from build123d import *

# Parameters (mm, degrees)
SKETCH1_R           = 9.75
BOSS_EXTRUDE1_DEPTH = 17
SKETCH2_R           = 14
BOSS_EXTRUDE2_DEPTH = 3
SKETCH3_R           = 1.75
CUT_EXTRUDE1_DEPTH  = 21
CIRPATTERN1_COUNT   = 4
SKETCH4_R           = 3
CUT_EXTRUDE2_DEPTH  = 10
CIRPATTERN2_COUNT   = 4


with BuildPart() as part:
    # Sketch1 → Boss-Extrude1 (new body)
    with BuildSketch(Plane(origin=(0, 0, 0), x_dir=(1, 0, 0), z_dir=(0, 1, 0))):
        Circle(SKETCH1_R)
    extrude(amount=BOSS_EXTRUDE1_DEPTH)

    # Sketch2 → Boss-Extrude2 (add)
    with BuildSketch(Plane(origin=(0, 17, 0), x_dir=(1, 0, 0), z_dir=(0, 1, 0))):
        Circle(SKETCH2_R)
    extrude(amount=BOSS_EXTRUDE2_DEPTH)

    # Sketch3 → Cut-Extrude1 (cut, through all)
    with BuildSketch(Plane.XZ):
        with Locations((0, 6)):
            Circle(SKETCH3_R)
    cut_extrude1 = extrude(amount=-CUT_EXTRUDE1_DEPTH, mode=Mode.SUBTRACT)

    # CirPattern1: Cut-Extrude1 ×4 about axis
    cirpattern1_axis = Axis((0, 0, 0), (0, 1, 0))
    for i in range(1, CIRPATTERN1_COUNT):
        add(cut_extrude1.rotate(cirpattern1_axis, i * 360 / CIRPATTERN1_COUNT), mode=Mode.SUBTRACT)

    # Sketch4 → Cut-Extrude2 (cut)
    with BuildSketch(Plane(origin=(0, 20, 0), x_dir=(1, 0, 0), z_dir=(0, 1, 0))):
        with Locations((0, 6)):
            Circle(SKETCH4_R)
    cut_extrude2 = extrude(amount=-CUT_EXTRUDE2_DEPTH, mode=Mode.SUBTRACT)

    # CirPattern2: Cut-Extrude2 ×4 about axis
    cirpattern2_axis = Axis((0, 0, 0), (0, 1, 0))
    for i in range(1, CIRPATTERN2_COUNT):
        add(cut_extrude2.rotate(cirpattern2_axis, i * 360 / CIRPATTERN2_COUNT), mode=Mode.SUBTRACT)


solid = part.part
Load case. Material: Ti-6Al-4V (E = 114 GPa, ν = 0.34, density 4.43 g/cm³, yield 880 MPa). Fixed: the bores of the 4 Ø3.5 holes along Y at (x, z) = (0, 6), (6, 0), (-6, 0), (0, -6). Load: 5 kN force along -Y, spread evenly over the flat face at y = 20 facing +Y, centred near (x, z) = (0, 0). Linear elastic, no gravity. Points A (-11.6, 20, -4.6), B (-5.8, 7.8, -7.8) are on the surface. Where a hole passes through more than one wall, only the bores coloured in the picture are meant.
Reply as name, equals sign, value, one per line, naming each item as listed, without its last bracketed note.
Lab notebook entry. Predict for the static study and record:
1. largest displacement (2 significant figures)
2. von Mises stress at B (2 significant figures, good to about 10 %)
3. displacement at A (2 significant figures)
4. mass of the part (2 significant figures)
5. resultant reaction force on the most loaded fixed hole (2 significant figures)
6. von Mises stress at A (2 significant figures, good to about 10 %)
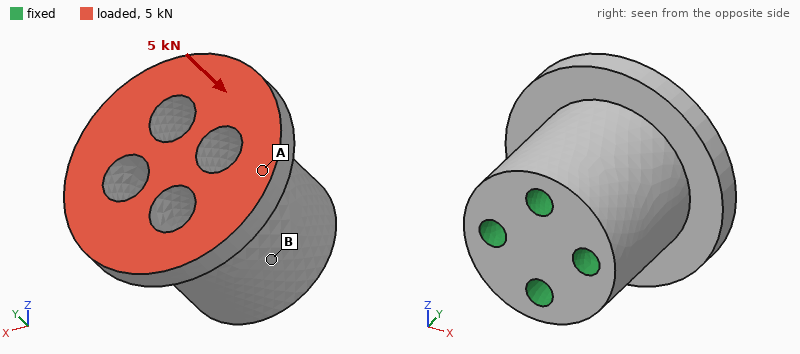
largest displacement = 14 µm
von Mises stress at B = 16 MPa
displacement at A = 11 µm
mass of the part = 24 g
resultant reaction force on the most loaded fixed hole = 1.3 kN
von Mises stress at A = 40 MPa
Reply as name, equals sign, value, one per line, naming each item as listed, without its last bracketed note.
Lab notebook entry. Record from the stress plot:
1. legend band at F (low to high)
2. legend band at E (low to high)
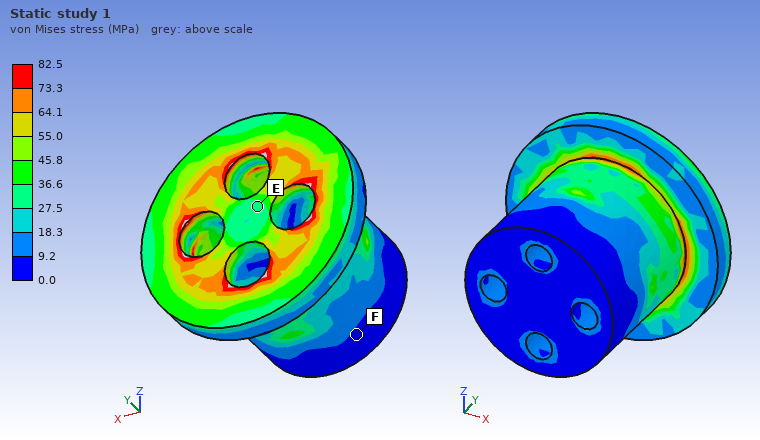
legend band at F = 0.0 to 9.2 MPa
legend band at E = 27.5 to 36.6 MPa
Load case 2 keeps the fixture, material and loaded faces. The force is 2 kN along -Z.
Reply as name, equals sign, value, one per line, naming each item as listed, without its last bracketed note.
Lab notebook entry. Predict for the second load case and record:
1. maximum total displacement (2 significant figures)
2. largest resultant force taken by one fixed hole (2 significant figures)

maximum total displacement = 14 µm
largest resultant force taken by one fixed hole = 1.4 kN
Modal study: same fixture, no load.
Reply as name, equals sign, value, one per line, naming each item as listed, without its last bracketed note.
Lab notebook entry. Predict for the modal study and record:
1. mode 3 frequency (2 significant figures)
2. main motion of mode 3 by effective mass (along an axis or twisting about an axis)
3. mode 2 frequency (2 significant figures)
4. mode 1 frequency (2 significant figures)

mode 3 frequency = 31 kHz
main motion of mode 3 by effective mass = twisting about Y
mode 2 frequency = 28 kHz
mode 1 frequency = 28 kHz
